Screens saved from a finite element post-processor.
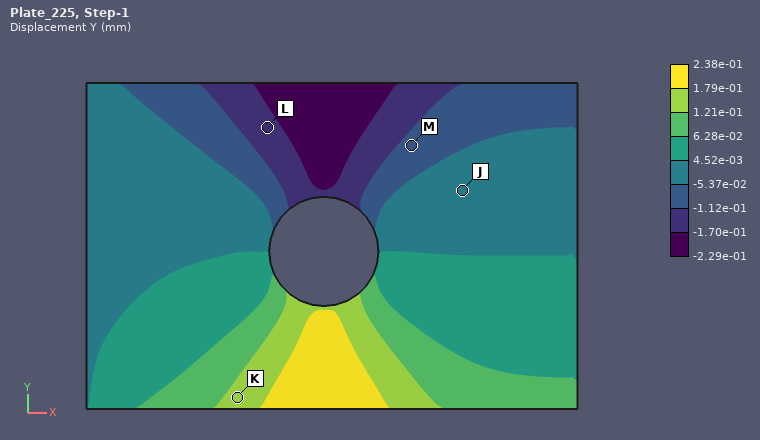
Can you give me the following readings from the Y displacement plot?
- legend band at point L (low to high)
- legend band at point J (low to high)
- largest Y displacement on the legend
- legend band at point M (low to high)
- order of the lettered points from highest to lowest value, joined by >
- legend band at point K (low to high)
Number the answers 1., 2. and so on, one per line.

1. -1.70e-01 to -1.12e-01 mm
2. -5.37e-02 to 4.52e-03 mm
3. 2.38e-01 mm
4. -1.12e-01 to -5.37e-02 mm
5. K > J > M > L
6. 1.21e-01 to 1.79e-01 mm
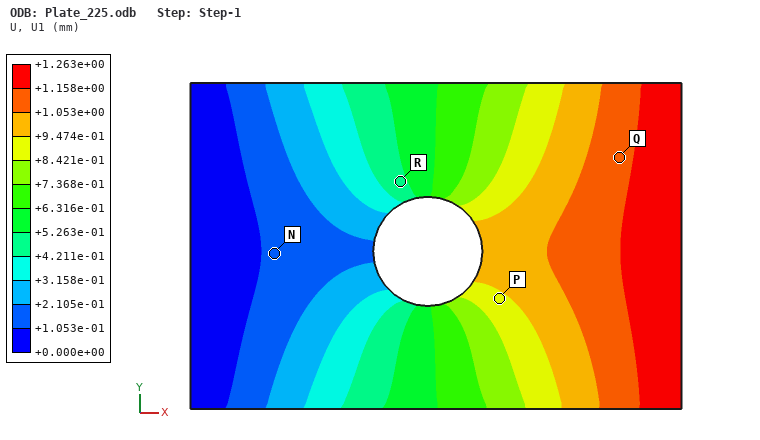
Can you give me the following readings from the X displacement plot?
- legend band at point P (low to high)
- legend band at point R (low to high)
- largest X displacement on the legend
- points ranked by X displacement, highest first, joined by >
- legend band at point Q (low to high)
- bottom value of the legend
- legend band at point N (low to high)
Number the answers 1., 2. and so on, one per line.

1. +8.421e-01 to +9.474e-01 mm
2. +4.211e-01 to +5.263e-01 mm
3. +1.263e+00 mm
4. Q > P > R > N
5. +1.053e+00 to +1.158e+00 mm
6. +0.000e+00 mm
7. +1.053e-01 to +2.105e-01 mm
